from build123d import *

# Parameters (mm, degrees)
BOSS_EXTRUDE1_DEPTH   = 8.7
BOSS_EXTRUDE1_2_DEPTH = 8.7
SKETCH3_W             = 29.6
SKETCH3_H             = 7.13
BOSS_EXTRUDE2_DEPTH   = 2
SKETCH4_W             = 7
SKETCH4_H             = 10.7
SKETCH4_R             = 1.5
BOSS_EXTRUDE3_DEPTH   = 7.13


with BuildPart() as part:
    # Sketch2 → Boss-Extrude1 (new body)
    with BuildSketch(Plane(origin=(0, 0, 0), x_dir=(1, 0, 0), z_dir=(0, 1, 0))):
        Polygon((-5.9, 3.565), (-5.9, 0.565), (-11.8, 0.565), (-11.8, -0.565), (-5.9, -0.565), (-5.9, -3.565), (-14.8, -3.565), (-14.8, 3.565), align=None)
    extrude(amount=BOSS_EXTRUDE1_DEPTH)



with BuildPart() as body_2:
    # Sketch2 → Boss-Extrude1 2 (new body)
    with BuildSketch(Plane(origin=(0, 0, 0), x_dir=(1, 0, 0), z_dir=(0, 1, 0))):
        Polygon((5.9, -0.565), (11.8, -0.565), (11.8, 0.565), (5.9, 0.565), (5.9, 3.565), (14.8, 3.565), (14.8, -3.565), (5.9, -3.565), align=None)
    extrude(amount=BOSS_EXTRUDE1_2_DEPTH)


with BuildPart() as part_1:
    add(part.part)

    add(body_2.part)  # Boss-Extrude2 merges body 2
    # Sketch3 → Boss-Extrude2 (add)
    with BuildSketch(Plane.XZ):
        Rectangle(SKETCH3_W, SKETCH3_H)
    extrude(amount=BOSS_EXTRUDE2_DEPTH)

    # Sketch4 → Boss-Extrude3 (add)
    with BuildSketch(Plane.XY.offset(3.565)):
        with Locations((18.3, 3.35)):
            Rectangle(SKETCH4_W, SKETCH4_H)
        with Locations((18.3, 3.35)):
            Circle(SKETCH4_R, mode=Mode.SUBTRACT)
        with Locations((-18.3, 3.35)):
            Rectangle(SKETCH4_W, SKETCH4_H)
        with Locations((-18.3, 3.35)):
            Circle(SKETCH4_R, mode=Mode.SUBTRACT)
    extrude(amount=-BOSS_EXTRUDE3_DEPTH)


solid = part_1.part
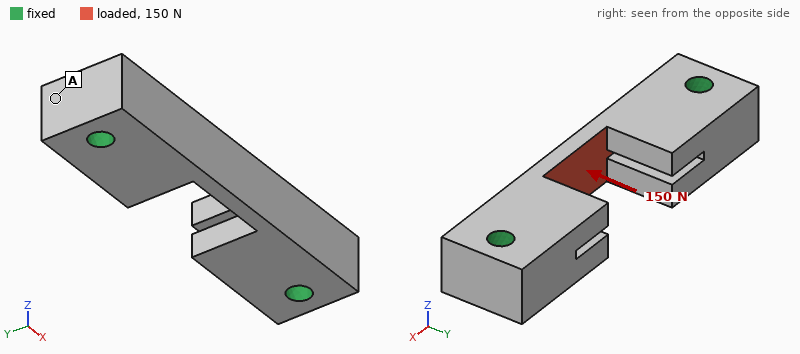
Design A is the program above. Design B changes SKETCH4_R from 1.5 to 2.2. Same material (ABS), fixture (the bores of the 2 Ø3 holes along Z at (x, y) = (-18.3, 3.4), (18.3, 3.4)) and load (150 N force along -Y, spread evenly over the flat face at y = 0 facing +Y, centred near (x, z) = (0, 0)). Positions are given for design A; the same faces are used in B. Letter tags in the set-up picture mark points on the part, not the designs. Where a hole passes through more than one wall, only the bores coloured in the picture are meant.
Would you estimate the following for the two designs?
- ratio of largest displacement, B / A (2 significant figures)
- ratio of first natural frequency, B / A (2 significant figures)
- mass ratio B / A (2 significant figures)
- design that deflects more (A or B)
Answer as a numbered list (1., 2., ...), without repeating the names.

1. 0.91
2. 1.1
3. 0.95
4. A
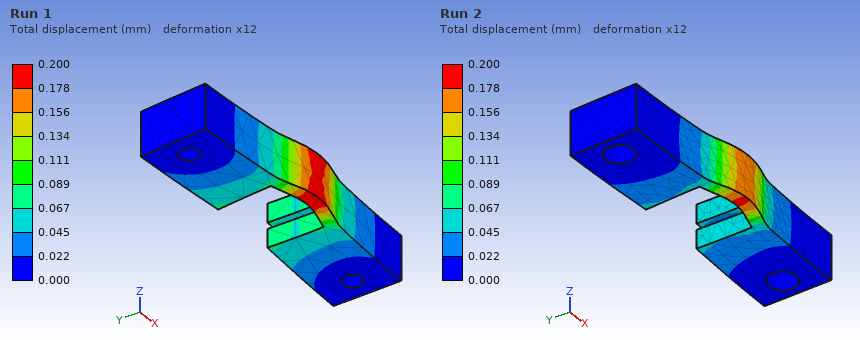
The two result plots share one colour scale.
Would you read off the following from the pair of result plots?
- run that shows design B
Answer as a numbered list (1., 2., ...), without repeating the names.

1. Run 2
